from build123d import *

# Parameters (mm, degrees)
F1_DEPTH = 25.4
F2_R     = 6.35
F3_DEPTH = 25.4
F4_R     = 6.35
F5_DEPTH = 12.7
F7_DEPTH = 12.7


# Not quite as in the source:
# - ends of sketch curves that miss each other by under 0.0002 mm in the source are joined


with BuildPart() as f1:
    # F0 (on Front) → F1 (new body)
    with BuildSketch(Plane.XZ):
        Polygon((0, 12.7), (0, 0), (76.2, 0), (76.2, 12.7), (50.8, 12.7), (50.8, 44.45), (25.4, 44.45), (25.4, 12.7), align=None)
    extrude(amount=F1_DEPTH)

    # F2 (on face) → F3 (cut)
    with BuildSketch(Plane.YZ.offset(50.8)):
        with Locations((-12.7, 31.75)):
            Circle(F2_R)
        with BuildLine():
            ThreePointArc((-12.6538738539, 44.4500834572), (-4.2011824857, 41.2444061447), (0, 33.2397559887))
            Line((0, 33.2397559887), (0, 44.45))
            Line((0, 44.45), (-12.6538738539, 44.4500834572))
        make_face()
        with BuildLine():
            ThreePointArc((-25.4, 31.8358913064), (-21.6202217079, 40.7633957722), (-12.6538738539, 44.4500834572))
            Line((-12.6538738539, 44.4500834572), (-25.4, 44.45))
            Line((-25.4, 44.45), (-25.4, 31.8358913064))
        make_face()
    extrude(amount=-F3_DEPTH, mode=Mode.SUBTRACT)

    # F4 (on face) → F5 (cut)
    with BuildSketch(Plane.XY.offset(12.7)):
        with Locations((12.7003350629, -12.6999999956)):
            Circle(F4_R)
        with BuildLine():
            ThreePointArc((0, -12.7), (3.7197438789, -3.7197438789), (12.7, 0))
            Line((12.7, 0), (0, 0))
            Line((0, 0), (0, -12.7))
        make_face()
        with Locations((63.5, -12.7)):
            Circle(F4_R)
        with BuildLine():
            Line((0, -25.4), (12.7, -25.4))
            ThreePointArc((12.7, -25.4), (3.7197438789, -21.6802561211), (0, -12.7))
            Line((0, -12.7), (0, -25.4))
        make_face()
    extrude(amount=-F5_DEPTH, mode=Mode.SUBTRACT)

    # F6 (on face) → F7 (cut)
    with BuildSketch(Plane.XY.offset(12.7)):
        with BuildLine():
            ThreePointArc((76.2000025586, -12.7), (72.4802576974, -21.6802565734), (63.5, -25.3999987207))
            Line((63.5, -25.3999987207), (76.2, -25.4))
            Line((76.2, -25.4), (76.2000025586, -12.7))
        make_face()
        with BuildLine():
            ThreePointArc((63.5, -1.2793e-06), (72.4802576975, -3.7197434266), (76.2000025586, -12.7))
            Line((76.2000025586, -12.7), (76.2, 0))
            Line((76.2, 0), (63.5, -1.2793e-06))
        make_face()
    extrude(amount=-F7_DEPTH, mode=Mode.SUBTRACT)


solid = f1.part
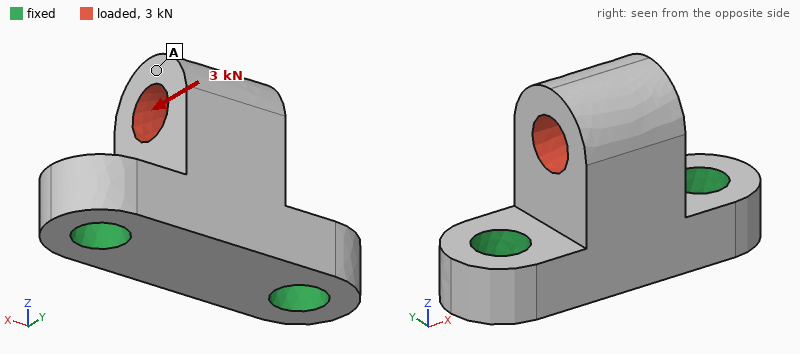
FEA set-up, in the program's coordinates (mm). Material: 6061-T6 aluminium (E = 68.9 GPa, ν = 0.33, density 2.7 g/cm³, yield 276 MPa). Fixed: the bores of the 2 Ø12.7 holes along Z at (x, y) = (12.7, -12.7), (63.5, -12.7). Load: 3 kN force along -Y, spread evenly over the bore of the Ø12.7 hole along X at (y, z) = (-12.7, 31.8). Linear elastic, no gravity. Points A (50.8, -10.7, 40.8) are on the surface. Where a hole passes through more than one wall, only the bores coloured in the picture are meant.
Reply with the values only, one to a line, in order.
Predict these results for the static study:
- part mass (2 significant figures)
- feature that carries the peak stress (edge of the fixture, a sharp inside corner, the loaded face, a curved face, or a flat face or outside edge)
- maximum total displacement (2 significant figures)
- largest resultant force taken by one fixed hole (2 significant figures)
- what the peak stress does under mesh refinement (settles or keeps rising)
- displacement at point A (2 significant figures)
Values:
95 g
edge of the fixture
65 µm
1.5 kN
keeps rising
60 µm
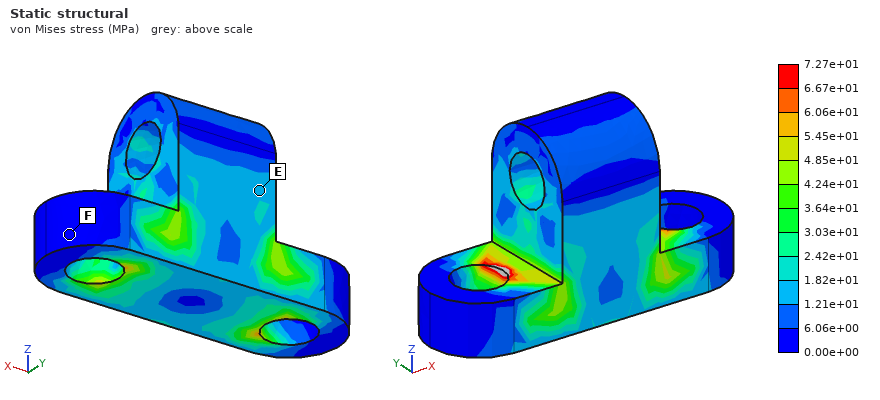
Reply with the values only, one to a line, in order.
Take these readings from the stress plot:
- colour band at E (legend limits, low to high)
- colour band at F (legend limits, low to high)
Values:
1.21e+01 to 1.82e+01 MPa
0.00e+00 to 6.06e+00 MPa
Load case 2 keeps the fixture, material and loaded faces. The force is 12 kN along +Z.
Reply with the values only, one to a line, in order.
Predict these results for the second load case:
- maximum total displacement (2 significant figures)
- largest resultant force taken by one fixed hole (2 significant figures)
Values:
27 µm
6.3 kN
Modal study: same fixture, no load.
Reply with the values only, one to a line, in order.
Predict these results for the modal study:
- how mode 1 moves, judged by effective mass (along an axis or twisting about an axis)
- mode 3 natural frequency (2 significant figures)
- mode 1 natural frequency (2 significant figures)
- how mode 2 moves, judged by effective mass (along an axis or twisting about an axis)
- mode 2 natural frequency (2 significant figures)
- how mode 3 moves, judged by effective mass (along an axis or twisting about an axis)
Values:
along Y
17 kHz
7000 Hz
along X
12 kHz
along Z
